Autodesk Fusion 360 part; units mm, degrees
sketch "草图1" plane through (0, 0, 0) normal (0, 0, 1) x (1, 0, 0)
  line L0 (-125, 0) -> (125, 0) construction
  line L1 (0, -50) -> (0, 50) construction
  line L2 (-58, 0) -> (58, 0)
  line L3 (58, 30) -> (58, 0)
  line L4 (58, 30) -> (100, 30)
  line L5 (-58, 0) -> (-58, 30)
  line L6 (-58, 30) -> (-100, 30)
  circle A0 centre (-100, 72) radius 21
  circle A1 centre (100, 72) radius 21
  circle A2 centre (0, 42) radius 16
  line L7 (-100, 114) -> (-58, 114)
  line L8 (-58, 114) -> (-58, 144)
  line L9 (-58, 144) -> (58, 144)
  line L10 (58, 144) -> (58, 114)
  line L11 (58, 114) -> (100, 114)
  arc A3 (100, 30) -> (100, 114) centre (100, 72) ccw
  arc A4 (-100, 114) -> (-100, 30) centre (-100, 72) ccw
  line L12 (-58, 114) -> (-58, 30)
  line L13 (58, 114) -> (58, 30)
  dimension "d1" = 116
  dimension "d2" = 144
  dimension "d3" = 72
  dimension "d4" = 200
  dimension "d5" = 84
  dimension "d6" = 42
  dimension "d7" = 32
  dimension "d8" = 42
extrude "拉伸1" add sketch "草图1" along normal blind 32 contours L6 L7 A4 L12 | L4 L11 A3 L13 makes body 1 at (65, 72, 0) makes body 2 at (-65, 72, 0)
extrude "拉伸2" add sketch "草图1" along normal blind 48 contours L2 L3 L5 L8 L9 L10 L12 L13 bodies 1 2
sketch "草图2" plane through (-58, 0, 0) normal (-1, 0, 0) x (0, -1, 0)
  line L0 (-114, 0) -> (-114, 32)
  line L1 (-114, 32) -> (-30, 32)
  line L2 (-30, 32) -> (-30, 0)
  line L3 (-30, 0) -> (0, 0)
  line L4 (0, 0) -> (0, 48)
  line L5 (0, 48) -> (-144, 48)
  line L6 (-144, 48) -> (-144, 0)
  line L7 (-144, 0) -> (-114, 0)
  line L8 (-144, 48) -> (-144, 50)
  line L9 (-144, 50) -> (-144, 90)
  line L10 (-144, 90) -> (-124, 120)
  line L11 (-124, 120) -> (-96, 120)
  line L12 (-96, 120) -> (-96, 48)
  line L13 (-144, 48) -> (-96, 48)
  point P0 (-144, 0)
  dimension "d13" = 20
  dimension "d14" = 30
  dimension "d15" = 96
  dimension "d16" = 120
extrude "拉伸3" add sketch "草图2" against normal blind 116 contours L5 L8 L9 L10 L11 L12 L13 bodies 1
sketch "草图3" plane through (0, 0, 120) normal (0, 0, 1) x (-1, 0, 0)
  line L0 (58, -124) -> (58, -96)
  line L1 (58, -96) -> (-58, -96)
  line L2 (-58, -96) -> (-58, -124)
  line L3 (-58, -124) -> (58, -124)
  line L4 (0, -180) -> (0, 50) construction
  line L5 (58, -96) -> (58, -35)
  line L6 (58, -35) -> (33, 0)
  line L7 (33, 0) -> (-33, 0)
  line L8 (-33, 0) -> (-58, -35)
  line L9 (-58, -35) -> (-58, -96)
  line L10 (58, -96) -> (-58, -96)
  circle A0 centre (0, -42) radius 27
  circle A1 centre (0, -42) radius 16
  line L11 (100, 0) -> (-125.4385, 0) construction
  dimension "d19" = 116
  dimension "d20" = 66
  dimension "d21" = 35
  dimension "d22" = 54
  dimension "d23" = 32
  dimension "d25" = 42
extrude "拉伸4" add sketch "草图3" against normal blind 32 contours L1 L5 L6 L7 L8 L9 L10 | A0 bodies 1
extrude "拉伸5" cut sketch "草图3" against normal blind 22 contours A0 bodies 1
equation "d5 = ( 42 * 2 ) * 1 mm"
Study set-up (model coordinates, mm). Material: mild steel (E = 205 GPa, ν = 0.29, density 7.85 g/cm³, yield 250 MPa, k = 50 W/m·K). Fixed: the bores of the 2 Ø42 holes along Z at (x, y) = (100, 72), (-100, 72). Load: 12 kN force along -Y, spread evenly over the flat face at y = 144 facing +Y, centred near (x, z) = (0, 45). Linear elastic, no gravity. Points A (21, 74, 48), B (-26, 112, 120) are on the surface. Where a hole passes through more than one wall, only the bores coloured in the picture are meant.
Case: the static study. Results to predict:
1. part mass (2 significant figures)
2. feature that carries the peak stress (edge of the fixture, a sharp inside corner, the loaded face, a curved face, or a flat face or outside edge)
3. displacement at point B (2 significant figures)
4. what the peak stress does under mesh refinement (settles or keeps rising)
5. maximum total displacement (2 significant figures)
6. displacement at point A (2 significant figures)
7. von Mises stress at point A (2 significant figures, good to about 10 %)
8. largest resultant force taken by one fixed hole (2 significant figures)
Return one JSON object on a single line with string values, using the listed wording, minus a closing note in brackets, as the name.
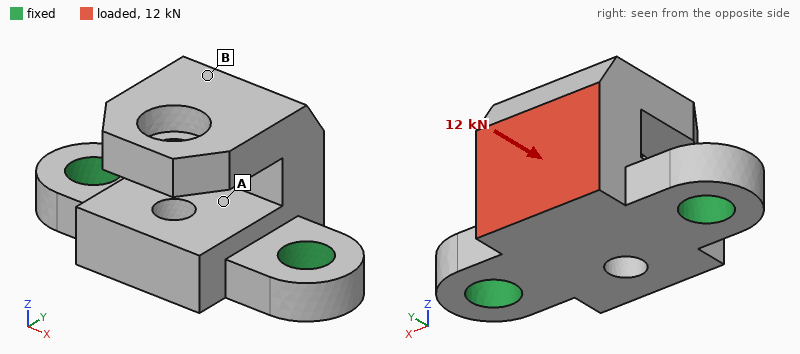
{"part mass": "13 kg", "feature that carries the peak stress": "edge of the fixture", "displacement at point B": "16 µm", "what the peak stress does under mesh refinement": "keeps rising", "maximum total displacement": "20 µm", "displacement at point A": "4.7 µm", "von Mises stress at point A": "4.4 MPa", "largest resultant force taken by one fixed hole": "6.1 kN"}
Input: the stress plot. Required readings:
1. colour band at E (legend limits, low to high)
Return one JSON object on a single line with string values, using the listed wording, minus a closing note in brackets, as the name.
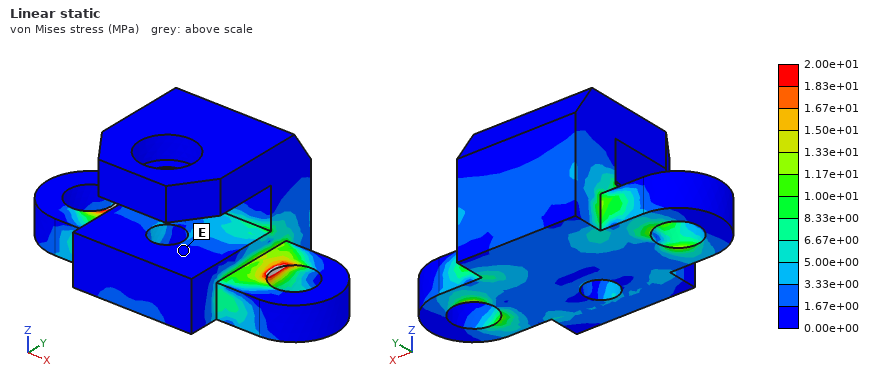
{"colour band at E": "0.00e+00 to 1.67e+00 MPa"}
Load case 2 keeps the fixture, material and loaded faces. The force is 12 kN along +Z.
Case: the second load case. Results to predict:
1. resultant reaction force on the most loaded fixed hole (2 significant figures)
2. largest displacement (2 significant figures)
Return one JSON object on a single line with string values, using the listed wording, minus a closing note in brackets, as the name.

{"resultant reaction force on the most loaded fixed hole": "6.6 kN", "largest displacement": "39 µm"}
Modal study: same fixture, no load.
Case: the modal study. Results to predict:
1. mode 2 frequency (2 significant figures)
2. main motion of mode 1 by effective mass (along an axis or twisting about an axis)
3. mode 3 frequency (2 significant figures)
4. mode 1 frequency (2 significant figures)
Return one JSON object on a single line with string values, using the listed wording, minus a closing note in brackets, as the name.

{"mode 2 frequency": "1900 Hz", "main motion of mode 1 by effective mass": "along Y", "mode 3 frequency": "2000 Hz", "mode 1 frequency": "1100 Hz"}
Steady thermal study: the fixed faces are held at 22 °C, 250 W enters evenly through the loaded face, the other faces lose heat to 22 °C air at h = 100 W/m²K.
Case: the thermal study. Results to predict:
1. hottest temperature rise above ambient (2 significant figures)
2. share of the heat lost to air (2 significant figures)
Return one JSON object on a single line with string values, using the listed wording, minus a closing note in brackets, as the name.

{"hottest temperature rise above ambient": "42 K", "share of the heat lost to air": "65 %"}
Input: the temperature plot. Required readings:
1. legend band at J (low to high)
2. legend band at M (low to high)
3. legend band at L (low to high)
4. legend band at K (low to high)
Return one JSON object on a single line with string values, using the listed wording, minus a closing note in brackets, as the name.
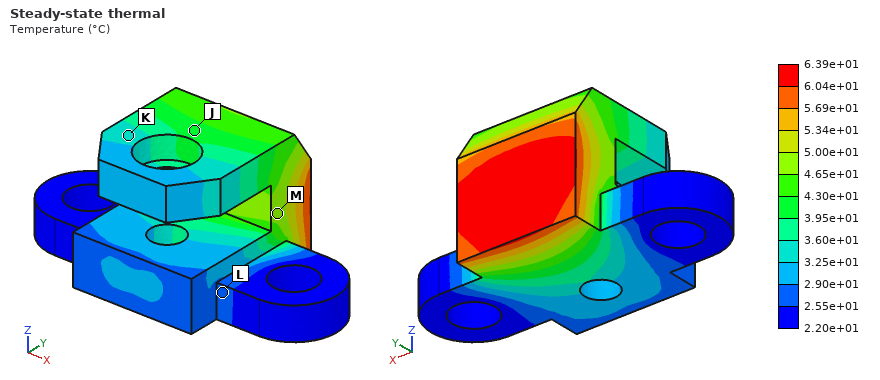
{"legend band at J": "3.95e+01 to 4.30e+01 °C", "legend band at M": "4.65e+01 to 5.00e+01 °C", "legend band at L": "2.55e+01 to 2.90e+01 °C", "legend band at K": "3.25e+01 to 3.60e+01 °C"}
